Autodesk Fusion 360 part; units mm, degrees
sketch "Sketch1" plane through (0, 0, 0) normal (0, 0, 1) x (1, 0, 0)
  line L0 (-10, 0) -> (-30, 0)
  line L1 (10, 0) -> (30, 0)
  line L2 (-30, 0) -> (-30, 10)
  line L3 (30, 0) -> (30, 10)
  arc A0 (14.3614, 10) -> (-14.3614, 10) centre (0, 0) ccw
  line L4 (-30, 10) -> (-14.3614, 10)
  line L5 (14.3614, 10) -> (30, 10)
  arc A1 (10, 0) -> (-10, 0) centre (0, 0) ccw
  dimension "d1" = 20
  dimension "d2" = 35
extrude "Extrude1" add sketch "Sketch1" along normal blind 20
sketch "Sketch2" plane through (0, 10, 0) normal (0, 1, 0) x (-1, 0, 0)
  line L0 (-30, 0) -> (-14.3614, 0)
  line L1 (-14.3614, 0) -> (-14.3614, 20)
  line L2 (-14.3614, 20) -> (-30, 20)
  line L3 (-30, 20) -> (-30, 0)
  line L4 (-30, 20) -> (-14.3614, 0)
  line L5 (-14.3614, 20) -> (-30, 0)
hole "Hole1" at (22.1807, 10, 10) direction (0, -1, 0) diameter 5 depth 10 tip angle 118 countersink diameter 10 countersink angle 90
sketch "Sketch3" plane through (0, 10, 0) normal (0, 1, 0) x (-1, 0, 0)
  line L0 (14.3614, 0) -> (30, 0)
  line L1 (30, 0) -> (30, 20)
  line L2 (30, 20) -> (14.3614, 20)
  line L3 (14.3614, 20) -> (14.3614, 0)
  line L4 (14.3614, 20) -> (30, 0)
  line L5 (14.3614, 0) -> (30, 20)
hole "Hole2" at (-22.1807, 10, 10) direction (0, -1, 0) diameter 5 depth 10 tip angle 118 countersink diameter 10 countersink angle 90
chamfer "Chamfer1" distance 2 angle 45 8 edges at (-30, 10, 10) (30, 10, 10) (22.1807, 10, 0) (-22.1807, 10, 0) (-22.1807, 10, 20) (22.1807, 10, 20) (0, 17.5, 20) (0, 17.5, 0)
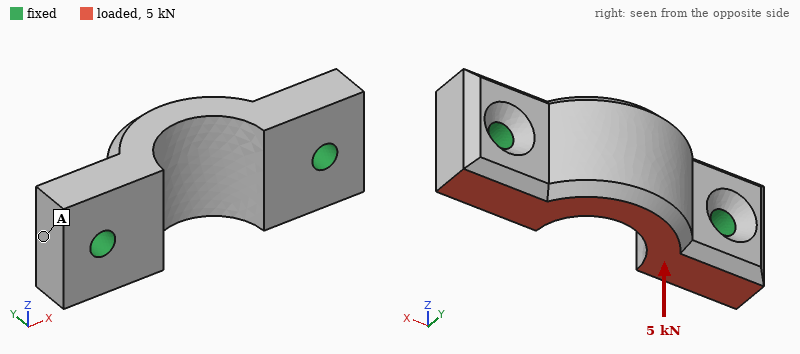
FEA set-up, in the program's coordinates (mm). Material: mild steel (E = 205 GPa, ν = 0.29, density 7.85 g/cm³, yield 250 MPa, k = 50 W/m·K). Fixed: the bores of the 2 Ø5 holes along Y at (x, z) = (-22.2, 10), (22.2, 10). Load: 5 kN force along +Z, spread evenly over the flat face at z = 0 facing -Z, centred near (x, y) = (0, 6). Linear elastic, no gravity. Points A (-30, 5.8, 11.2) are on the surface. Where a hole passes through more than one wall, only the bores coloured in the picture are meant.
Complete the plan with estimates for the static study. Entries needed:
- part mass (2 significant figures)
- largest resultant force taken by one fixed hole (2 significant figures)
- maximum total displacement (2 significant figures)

87 g
2.5 kN
7.4 µm
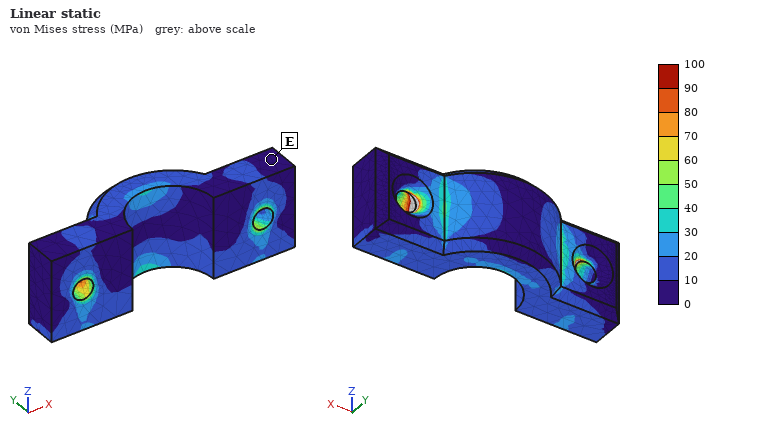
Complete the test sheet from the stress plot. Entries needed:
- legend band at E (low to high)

0 to 10 MPa
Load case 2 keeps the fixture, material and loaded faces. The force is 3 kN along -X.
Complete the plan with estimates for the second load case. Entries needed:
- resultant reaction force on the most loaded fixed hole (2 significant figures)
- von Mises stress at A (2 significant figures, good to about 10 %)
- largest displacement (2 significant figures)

1.6 kN
10 MPa
2.4 µm
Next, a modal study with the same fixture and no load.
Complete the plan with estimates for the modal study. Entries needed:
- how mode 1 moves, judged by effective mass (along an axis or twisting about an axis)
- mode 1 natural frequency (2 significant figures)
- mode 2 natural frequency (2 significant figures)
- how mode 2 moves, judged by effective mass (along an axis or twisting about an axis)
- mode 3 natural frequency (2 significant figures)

along Z
15 kHz
23 kHz
along Y
30 kHz
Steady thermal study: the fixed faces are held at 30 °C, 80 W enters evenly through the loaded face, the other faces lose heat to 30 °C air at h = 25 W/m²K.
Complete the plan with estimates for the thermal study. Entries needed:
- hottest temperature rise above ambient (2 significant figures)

60 K
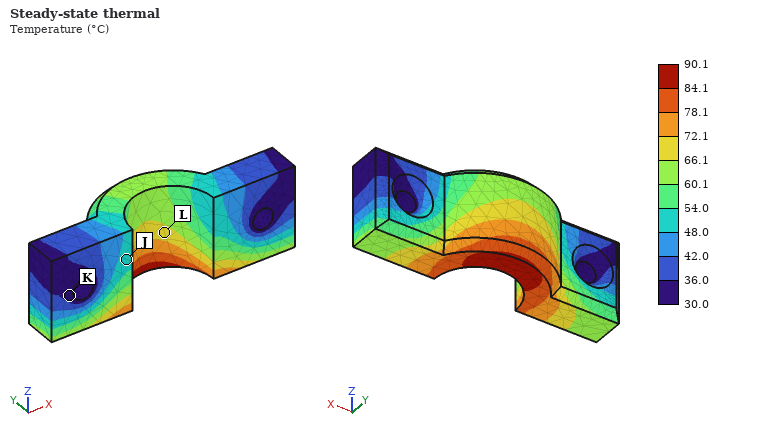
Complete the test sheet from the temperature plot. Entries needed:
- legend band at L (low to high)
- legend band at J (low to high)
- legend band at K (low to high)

66.1 to 72.1 °C
48.0 to 54.0 °C
30.0 to 36.0 °C
